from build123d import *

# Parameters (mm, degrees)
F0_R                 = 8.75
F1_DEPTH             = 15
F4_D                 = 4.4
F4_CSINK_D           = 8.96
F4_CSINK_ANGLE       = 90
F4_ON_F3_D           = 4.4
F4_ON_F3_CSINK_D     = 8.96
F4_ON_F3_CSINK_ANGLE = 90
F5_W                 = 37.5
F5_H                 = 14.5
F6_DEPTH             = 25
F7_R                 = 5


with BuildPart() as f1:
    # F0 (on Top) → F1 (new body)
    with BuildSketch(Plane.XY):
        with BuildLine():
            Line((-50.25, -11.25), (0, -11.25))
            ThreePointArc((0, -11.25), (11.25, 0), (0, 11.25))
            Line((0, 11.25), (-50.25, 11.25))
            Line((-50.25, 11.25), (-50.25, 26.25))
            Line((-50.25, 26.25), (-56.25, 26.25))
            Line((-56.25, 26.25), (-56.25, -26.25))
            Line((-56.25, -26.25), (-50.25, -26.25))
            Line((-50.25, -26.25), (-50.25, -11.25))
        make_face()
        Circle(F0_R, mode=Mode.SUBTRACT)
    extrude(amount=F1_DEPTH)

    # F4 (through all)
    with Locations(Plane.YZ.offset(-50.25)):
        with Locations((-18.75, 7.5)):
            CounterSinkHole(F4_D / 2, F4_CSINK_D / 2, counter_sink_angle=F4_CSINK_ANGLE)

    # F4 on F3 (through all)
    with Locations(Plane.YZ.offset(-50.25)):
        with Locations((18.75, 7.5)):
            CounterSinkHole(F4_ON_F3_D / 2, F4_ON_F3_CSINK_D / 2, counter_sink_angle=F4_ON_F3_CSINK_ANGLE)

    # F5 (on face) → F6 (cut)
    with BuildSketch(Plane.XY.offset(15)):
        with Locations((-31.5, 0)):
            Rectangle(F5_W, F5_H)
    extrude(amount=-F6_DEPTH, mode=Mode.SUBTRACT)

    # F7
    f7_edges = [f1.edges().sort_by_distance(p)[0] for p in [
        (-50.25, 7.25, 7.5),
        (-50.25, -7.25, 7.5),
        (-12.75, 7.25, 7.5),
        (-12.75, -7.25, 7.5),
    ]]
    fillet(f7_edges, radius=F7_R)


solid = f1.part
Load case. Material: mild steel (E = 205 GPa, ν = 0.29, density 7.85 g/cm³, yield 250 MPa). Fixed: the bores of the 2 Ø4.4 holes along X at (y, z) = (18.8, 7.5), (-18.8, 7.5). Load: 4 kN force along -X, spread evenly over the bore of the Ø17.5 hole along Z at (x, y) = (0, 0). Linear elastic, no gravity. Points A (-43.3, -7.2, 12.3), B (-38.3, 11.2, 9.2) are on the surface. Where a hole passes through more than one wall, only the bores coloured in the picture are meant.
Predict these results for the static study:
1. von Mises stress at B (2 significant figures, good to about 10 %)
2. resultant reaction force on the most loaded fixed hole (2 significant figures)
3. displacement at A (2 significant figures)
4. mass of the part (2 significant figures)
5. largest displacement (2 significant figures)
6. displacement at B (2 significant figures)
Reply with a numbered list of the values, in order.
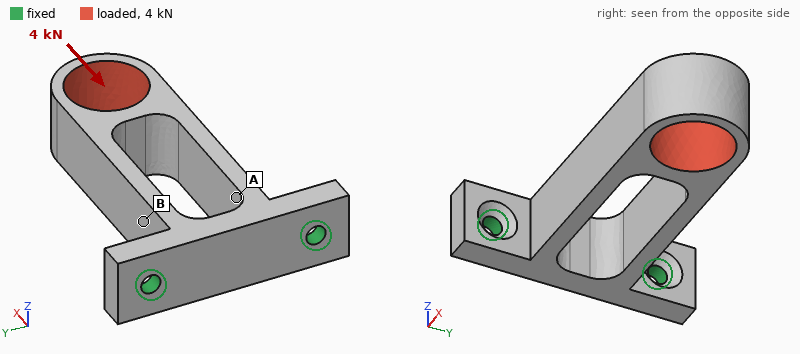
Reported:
1. 49 MPa
2. 2.3 kN
3. 13 µm
4. 100 g
5. 26 µm
6. 13 µm
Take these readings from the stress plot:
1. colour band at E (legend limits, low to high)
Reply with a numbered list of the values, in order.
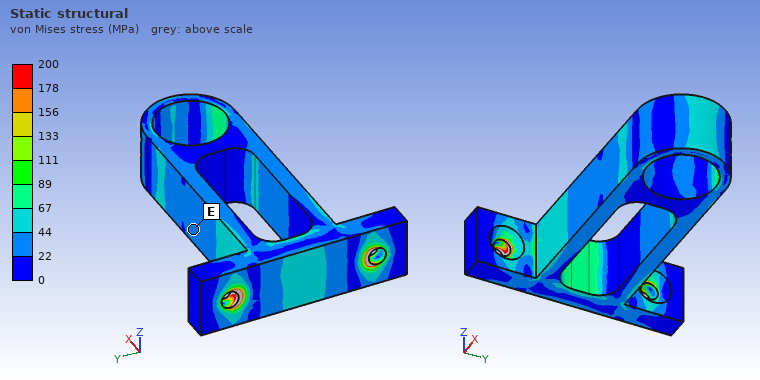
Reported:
1. 22 to 44 MPa
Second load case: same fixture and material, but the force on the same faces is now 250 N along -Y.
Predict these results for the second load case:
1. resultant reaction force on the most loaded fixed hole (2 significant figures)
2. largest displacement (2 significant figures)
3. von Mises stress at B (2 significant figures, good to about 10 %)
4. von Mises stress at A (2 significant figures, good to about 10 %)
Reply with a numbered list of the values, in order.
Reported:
1. 450 N
2. 47 µm
3. 29 MPa
4. 32 MPa
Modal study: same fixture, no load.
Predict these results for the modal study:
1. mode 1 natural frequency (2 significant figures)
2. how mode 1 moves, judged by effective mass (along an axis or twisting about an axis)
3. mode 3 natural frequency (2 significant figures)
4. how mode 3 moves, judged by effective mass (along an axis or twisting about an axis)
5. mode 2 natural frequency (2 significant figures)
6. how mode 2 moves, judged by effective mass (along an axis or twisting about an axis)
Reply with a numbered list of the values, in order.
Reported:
1. 1500 Hz
2. along Z
3. 4800 Hz
4. twisting about X
5. 2000 Hz
6. along Y
